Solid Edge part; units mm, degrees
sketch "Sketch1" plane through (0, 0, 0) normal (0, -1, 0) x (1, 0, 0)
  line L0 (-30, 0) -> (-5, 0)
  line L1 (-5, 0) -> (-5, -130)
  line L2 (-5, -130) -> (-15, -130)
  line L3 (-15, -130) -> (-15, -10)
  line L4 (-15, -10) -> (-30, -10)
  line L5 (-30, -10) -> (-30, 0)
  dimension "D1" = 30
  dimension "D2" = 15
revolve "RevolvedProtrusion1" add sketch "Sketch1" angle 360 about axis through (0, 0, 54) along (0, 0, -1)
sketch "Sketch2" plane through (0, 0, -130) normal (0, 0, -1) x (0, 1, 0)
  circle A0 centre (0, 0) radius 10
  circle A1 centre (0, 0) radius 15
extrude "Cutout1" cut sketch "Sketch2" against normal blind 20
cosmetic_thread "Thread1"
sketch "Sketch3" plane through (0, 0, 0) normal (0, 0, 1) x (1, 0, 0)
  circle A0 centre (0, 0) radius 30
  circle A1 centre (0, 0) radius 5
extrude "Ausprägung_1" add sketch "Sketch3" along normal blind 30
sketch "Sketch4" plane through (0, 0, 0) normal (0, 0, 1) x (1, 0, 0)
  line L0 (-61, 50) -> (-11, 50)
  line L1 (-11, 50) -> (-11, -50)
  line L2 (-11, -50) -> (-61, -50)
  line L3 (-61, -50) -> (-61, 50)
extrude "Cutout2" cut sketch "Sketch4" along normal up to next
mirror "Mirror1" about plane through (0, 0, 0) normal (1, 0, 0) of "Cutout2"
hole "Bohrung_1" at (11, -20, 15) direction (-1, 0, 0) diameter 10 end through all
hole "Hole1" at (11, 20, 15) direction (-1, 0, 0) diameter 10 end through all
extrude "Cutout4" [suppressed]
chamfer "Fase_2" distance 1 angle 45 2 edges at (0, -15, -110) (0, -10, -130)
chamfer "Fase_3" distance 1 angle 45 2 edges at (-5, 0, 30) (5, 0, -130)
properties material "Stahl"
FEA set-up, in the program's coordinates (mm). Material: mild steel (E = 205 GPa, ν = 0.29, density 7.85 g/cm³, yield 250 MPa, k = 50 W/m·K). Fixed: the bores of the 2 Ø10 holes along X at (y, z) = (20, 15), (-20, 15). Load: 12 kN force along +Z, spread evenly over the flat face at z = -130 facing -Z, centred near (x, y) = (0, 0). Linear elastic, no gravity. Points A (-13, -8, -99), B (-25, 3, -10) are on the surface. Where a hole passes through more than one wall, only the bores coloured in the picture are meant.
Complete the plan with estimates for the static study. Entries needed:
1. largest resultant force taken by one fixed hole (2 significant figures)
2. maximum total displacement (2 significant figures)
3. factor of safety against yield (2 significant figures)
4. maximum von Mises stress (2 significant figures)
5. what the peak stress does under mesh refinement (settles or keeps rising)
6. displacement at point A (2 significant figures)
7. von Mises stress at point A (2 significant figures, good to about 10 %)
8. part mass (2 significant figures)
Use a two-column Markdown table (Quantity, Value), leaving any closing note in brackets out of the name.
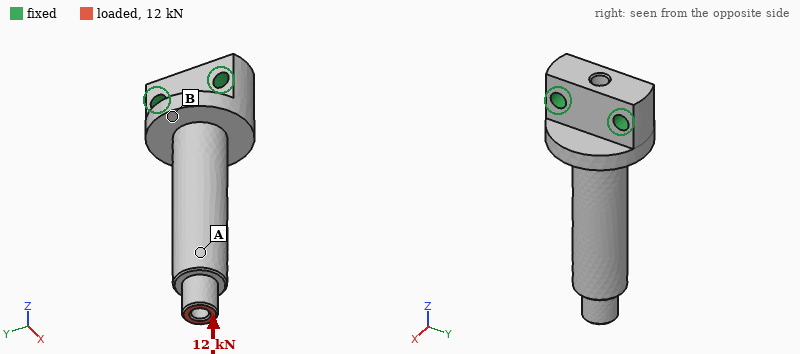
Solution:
| Quantity | Value |
|---|---|
| largest resultant force taken by one fixed hole | 6.3 kN |
| maximum total displacement | 17 µm |
| factor of safety against yield | 3.4 |
| maximum von Mises stress | 75 MPa |
| what the peak stress does under mesh refinement | settles |
| displacement at point A | 10 µm |
| von Mises stress at point A | 16 MPa |
| part mass | 1.0 kg |
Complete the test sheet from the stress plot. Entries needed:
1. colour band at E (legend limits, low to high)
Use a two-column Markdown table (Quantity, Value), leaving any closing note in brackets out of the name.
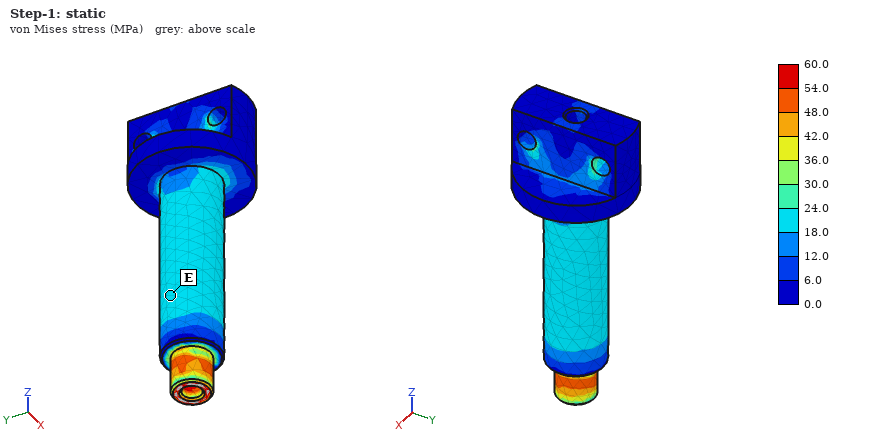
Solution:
| Quantity | Value |
|---|---|
| colour band at E | 18.0 to 24.0 MPa |
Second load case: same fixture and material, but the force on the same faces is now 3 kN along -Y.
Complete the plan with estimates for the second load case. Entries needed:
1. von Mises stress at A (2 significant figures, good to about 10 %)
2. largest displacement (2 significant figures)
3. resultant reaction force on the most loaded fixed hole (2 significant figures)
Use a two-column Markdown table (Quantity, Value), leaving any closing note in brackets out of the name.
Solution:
| Quantity | Value |
|---|---|
| von Mises stress at A | 19 MPa |
| largest displacement | 0.28 mm |
| resultant reaction force on the most loaded fixed hole | 11 kN |
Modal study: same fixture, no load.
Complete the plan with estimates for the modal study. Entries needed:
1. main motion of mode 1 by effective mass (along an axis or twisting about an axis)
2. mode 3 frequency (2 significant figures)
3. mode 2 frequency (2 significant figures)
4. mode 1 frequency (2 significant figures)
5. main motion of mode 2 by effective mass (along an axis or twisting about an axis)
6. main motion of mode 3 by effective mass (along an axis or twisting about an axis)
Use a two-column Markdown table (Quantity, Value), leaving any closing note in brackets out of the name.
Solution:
| Quantity | Value |
|---|---|
| main motion of mode 1 by effective mass | along X |
| mode 3 frequency | 6400 Hz |
| mode 2 frequency | 1600 Hz |
| mode 1 frequency | 1300 Hz |
| main motion of mode 2 by effective mass | along Y |
| main motion of mode 3 by effective mass | along X |
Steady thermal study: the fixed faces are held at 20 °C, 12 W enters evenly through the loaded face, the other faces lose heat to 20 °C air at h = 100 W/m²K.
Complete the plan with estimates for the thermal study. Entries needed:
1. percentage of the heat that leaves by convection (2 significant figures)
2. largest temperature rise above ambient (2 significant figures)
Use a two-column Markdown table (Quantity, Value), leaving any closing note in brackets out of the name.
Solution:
| Quantity | Value |
|---|---|
| percentage of the heat that leaves by convection | 89 % |
| largest temperature rise above ambient | 30 K |
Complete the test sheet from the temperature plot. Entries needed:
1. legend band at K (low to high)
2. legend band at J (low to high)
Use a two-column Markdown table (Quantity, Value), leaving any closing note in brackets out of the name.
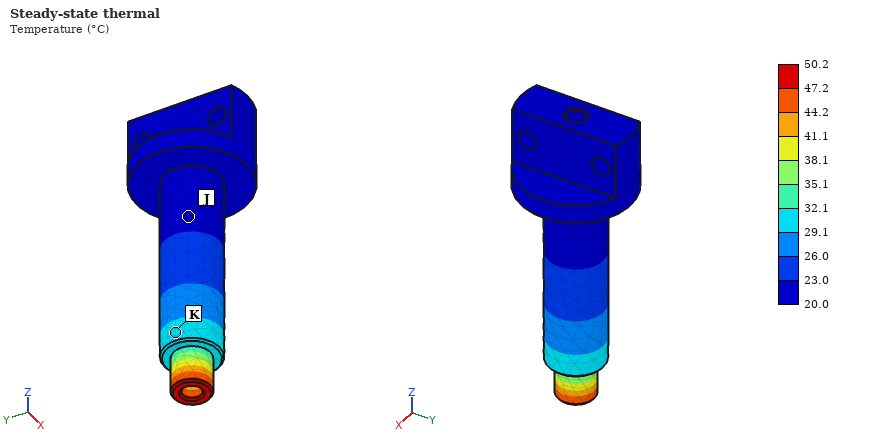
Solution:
| Quantity | Value |
|---|---|
| legend band at K | 29.1 to 32.1 °C |
| legend band at J | 20.0 to 23.0 °C |
